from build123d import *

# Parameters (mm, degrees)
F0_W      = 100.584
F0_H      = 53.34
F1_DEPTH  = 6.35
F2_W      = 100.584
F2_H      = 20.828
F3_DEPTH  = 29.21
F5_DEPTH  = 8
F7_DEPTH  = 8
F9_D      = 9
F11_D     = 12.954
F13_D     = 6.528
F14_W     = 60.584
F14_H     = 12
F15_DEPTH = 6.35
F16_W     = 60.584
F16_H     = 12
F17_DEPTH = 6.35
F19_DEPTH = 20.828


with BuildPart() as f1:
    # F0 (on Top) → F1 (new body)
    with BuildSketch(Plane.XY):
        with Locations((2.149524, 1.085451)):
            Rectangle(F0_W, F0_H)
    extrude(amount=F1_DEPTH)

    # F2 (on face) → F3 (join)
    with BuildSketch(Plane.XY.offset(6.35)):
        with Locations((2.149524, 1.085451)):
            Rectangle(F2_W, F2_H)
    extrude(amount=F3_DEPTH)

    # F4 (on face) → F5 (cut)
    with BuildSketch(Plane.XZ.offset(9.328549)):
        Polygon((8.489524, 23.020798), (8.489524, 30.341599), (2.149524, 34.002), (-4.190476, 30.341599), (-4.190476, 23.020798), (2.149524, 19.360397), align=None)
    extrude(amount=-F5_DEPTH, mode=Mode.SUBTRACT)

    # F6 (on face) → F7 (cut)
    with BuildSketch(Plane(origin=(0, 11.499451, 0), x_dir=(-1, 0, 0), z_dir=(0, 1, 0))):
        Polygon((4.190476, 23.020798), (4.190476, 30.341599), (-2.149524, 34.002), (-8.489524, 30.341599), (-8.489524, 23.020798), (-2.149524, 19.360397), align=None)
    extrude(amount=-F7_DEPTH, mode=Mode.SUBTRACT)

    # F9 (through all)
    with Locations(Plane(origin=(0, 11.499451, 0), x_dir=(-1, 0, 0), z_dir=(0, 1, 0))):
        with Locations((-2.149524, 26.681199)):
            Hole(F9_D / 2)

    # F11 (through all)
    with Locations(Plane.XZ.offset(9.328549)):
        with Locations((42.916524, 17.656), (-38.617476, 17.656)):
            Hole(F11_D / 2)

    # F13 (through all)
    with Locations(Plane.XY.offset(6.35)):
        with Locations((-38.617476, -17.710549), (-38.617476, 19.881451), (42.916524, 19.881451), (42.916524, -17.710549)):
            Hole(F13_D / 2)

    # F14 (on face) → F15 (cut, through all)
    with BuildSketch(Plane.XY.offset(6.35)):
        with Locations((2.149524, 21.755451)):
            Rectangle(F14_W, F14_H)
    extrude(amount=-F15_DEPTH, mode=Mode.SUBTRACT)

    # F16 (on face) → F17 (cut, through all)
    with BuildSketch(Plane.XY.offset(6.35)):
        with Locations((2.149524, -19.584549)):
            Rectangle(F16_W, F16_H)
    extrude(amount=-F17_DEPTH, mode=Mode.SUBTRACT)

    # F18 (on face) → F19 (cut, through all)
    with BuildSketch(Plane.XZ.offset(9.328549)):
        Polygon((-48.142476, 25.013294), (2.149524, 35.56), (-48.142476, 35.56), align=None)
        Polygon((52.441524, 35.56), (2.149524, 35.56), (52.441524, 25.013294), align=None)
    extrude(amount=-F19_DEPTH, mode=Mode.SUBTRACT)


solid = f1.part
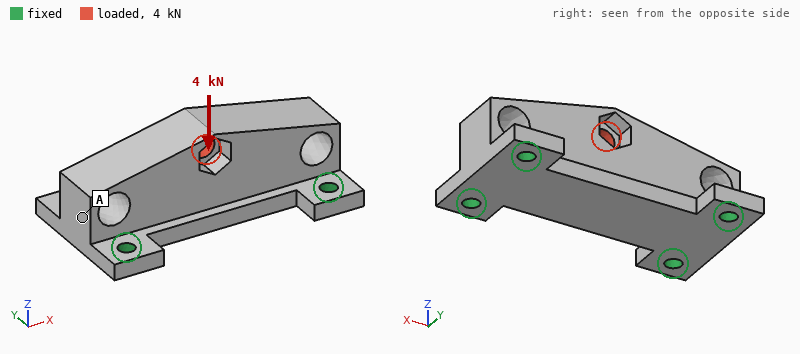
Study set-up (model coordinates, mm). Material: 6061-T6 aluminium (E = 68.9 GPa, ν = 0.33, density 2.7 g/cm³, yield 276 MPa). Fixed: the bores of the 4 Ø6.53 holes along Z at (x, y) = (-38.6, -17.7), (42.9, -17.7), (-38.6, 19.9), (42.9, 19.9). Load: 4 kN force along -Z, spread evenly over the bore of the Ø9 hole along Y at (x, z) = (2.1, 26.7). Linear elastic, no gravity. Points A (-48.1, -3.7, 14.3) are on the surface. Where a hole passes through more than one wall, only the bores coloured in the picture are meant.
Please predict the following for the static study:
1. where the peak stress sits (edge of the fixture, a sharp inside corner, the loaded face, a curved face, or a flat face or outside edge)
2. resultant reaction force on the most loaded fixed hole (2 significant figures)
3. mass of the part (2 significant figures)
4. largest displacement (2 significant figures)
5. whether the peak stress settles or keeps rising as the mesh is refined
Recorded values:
edge of the fixture
1.3 kN
180 g
23 µm
keeps rising
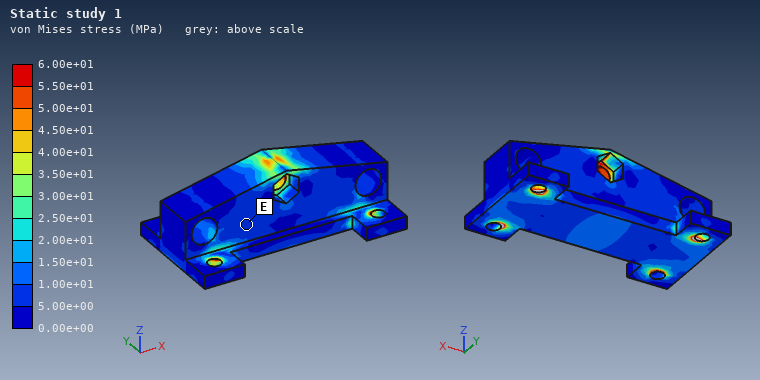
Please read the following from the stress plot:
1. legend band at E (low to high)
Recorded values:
5.00e+00 to 1.00e+01 MPa
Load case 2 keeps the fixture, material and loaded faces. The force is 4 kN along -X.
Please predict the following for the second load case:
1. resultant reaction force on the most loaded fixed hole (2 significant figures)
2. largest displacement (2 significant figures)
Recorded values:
1.2 kN
13 µm
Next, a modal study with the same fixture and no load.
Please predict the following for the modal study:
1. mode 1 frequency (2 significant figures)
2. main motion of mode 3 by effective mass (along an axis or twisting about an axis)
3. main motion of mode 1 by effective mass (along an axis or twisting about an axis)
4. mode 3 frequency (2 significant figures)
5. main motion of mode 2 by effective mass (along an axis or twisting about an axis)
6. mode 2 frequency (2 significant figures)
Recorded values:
6600 Hz
along X
along Y
11 kHz
along Z
7300 Hz
